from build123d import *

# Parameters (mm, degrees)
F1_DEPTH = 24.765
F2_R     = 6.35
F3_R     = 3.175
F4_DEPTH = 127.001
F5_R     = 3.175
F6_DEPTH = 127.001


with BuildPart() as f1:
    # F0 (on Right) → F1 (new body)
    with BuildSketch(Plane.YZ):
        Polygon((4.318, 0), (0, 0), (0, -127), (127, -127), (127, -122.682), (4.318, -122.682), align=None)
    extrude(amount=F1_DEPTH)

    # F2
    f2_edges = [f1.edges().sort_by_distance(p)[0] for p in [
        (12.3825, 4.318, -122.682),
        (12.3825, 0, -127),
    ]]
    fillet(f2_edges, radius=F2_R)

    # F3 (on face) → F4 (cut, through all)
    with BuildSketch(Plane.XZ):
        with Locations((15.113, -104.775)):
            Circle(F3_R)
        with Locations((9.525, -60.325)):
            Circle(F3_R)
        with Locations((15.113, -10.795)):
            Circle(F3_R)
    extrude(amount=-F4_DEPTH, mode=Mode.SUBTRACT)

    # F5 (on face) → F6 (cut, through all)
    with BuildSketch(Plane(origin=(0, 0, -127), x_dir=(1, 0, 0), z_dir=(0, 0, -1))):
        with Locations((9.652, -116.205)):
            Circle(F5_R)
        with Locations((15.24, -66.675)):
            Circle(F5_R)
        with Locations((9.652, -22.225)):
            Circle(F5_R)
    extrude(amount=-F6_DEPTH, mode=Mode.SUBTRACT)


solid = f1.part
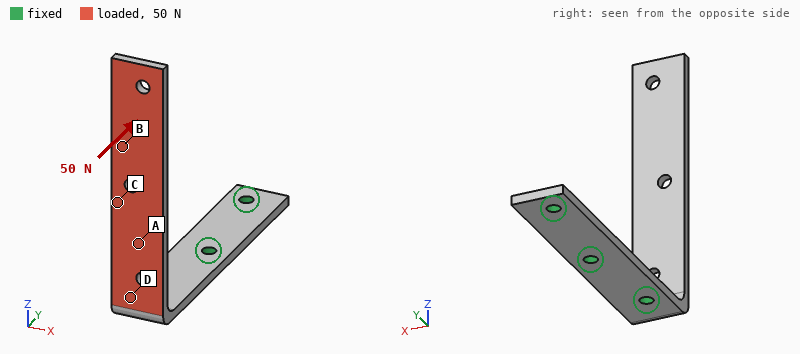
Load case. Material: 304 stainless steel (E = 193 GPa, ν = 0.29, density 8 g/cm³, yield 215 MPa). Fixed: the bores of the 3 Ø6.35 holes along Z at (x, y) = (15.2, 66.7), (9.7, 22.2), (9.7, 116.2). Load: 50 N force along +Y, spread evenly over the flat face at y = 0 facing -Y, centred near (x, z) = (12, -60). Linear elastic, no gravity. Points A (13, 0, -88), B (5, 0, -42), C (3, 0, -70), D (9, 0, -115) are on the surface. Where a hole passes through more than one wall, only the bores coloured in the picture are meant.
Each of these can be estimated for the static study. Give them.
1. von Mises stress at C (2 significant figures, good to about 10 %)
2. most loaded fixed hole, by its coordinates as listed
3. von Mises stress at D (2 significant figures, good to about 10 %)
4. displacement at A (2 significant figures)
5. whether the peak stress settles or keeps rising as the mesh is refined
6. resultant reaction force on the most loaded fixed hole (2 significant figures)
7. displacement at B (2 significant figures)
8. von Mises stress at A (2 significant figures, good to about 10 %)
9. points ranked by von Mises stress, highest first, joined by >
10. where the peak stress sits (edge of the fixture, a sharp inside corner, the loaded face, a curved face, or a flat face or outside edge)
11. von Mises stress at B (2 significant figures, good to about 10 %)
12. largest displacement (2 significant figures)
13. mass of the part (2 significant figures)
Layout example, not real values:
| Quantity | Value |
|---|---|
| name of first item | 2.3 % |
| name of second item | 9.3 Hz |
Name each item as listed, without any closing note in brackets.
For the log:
| Quantity | Value |
|---|---|
| von Mises stress at C | 13 MPa |
| most loaded fixed hole, by its coordinates as listed | (9.7, 22.2) |
| von Mises stress at D | 32 MPa |
| displacement at A | 0.10 mm |
| whether the peak stress settles or keeps rising as the mesh is refined | keeps rising |
| resultant reaction force on the most loaded fixed hole | 47 N |
| displacement at B | 0.32 mm |
| von Mises stress at A | 21 MPa |
| points ranked by von Mises stress, highest first, joined by > | D > A > C > B |
| where the peak stress sits | edge of the fixture |
| von Mises stress at B | 4.8 MPa |
| largest displacement | 0.55 mm |
| mass of the part | 210 g |
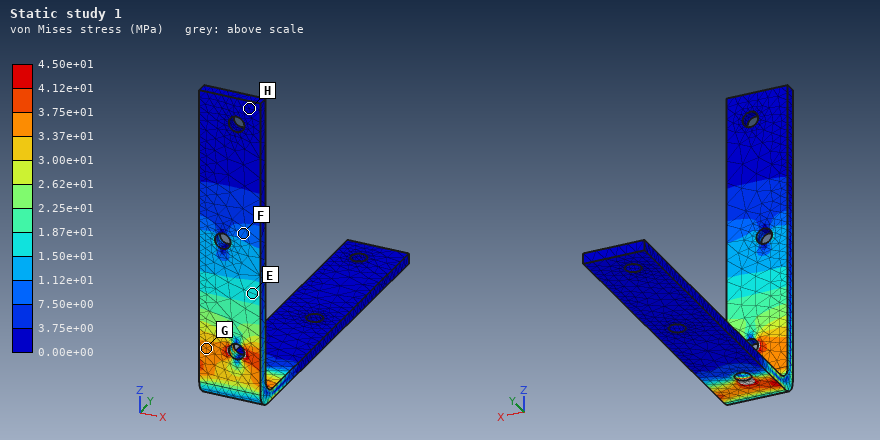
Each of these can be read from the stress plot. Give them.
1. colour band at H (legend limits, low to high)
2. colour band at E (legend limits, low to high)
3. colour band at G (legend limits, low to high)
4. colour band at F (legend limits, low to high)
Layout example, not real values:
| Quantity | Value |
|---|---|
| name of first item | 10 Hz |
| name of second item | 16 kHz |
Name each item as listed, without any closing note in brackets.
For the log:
| Quantity | Value |
|---|---|
| colour band at H | 0.00e+00 to 3.75e+00 MPa |
| colour band at E | 1.50e+01 to 1.87e+01 MPa |
| colour band at G | 3.37e+01 to 3.75e+01 MPa |
| colour band at F | 7.50e+00 to 1.12e+01 MPa |
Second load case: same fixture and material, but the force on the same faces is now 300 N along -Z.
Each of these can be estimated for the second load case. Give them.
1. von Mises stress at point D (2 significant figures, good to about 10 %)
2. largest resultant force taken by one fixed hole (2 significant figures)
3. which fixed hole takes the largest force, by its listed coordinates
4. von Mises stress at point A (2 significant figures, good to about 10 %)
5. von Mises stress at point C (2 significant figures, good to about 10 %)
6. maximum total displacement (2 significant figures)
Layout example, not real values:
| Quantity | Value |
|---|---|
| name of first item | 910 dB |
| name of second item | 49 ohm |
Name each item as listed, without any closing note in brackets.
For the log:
| Quantity | Value |
|---|---|
| von Mises stress at point D | 10 MPa |
| largest resultant force taken by one fixed hole | 310 N |
| which fixed hole takes the largest force, by its listed coordinates | (9.7, 22.2) |
| von Mises stress at point A | 8.0 MPa |
| von Mises stress at point C | 6.8 MPa |
| maximum total displacement | 0.35 mm |
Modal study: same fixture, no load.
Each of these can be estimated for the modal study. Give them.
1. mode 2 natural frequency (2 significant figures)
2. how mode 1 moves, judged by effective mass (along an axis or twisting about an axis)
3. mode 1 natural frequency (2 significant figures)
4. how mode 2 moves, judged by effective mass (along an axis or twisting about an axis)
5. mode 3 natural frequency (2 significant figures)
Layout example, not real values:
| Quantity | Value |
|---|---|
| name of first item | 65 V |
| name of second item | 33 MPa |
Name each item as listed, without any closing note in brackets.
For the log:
| Quantity | Value |
|---|---|
| mode 2 natural frequency | 390 Hz |
| how mode 1 moves, judged by effective mass | along Y |
| mode 1 natural frequency | 190 Hz |
| how mode 2 moves, judged by effective mass | along X |
| mode 3 natural frequency | 1200 Hz |
